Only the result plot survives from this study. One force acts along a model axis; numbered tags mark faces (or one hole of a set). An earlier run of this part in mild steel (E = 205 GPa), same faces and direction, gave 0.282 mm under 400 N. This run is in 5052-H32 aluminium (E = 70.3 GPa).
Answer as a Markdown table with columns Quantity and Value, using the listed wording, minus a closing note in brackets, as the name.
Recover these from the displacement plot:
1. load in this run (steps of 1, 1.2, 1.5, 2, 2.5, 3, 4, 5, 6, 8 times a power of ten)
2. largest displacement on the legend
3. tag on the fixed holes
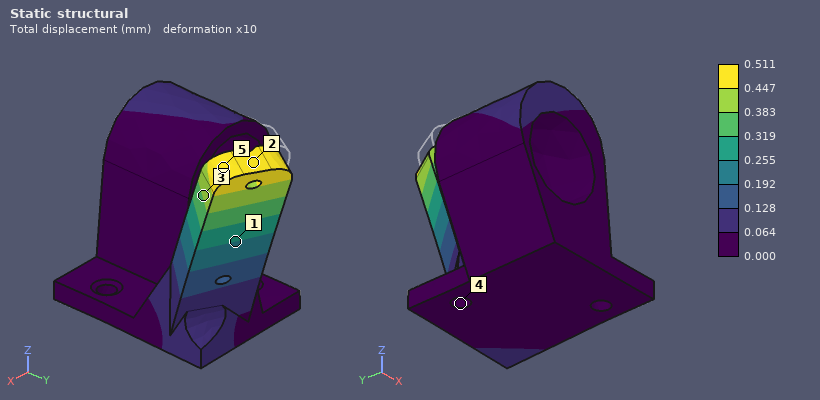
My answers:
| Quantity | Value |
|---|---|
| load in this run | 250 N |
| largest displacement on the legend | 0.511 mm |
| tag on the fixed holes | 4 |
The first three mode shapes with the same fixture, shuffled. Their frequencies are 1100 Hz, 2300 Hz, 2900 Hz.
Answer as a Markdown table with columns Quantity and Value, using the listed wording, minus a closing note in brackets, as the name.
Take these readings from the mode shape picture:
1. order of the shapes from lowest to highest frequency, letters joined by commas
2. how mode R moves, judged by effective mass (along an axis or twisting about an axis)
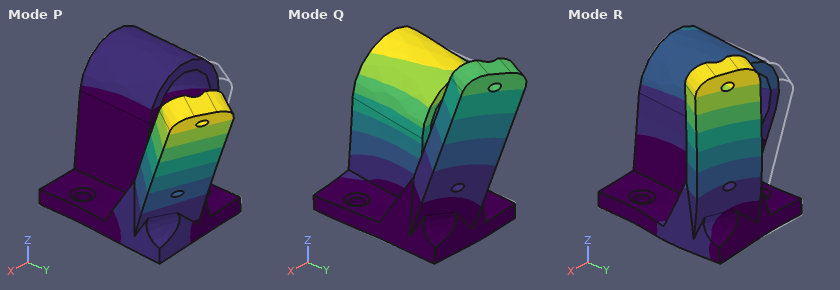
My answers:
| Quantity | Value |
|---|---|
| order of the shapes from lowest to highest frequency, letters joined by commas | P, R, Q |
| how mode R moves, judged by effective mass | along X |
